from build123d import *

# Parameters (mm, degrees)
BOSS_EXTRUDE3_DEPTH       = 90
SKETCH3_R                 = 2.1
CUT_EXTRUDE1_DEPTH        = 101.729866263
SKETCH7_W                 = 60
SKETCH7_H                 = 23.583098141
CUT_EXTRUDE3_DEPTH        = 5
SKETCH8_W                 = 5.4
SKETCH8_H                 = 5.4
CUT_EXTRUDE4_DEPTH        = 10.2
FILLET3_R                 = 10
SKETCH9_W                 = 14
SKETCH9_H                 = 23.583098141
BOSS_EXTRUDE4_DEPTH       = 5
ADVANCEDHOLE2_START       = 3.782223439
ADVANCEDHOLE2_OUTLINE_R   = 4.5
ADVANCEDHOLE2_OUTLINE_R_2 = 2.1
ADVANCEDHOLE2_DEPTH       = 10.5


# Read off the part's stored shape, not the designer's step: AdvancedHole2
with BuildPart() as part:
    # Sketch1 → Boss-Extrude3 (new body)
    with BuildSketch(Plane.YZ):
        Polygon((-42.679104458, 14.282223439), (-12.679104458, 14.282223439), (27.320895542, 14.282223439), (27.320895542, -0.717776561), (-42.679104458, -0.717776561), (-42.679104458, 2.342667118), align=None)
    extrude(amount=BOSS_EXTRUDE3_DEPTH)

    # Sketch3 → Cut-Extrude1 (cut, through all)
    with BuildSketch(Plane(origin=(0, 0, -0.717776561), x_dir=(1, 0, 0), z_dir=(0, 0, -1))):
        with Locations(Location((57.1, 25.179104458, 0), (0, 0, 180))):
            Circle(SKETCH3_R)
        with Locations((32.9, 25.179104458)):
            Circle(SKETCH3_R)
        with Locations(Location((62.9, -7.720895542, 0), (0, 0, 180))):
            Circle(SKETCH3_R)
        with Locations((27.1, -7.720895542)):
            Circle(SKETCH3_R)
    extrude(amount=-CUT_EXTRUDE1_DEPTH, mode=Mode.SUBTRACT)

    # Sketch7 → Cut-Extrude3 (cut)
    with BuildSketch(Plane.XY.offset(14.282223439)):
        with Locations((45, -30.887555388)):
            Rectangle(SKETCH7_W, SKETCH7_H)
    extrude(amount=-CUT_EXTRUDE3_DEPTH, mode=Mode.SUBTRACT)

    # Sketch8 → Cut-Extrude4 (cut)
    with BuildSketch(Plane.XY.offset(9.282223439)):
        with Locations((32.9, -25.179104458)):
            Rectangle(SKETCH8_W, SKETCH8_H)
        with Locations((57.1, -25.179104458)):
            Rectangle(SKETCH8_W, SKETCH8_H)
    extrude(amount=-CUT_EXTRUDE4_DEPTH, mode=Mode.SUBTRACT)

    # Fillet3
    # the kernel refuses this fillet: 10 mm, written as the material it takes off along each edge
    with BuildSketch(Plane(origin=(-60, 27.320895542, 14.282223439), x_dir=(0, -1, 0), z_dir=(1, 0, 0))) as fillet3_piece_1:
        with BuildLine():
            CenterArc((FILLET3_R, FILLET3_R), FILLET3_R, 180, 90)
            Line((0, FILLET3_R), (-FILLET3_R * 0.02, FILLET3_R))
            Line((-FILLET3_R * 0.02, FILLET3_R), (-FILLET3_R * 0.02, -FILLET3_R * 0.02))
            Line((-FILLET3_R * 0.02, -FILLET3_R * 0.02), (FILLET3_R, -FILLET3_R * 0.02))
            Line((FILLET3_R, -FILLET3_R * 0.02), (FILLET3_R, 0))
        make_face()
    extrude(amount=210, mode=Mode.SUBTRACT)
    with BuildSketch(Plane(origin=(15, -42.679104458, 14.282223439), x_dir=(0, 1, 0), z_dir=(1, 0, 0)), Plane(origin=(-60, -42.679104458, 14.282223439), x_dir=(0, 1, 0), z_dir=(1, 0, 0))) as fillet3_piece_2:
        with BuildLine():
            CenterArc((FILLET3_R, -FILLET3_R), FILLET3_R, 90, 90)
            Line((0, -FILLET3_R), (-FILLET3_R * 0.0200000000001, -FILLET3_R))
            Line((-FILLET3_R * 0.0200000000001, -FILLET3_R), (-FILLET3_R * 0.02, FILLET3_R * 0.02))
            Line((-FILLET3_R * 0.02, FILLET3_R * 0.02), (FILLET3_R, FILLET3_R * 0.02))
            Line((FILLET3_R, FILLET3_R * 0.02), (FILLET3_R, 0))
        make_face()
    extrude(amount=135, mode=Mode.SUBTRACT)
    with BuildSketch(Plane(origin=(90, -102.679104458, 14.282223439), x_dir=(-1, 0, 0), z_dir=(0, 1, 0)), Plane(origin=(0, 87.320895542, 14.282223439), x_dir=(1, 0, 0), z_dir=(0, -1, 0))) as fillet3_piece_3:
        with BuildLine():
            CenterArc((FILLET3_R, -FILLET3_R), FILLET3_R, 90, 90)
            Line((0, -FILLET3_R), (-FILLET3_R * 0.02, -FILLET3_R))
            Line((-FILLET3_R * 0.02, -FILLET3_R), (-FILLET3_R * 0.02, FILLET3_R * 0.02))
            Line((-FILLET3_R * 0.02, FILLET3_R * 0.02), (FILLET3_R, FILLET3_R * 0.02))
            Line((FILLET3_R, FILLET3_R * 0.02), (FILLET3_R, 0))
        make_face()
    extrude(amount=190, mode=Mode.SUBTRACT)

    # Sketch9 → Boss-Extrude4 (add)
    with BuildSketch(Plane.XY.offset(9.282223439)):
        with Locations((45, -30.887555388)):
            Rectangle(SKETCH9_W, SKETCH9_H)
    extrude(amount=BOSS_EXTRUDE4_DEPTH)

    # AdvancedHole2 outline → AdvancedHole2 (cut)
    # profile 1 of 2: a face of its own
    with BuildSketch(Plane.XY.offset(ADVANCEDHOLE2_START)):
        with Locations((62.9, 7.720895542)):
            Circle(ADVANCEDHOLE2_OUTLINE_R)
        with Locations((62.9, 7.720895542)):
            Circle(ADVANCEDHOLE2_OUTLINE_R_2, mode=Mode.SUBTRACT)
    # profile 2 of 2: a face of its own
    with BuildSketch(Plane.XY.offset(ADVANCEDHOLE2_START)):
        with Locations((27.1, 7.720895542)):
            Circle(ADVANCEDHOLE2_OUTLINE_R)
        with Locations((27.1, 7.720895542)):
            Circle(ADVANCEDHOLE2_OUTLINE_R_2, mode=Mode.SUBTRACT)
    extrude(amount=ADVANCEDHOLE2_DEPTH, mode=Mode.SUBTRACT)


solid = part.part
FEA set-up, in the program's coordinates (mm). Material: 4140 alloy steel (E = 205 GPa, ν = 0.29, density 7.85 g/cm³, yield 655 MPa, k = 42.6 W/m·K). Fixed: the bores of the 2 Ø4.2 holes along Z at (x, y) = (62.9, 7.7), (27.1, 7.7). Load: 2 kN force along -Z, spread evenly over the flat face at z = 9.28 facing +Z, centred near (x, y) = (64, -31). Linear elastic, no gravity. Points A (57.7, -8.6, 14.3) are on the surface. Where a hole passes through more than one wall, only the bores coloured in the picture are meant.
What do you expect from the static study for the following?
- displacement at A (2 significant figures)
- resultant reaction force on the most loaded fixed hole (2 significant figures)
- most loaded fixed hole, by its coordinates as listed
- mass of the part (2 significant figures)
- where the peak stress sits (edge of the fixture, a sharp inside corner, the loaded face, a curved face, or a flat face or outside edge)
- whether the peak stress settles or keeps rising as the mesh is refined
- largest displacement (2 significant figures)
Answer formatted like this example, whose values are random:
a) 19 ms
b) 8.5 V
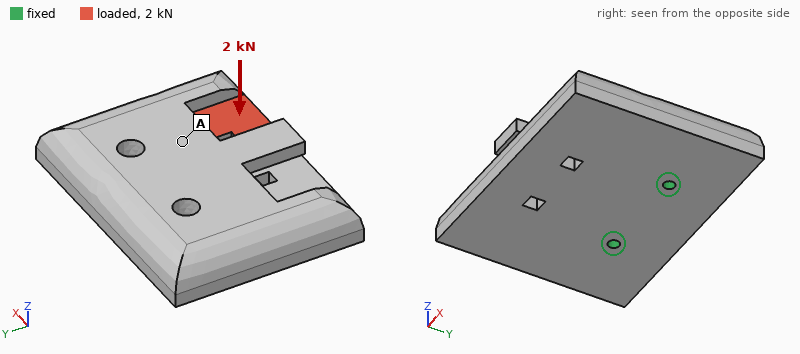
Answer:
a) 0.055 mm
b) 2.0 kN
c) (62.9, 7.7)
d) 640 g
e) edge of the fixture
f) keeps rising
g) 0.15 mm
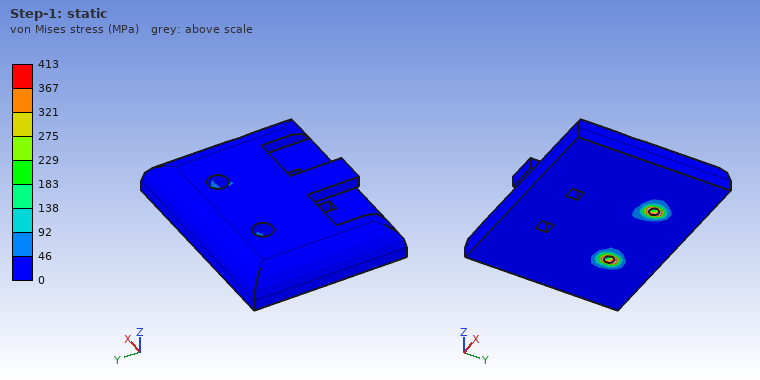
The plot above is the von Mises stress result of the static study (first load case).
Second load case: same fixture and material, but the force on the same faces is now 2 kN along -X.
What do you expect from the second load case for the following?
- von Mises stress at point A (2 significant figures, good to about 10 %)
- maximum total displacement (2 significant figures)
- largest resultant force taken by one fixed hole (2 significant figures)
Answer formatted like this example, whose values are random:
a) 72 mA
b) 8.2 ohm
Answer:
a) 7.3 MPa
b) 7.5 µm
c) 2.4 kN
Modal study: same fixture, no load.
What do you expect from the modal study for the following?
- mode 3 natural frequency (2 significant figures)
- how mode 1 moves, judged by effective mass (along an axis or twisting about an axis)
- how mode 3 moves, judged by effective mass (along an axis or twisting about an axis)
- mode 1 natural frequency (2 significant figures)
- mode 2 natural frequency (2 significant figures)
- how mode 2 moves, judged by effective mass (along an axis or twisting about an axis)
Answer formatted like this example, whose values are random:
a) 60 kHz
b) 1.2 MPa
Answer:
a) 5500 Hz
b) along Z
c) along X
d) 1400 Hz
e) 4200 Hz
f) twisting about Y
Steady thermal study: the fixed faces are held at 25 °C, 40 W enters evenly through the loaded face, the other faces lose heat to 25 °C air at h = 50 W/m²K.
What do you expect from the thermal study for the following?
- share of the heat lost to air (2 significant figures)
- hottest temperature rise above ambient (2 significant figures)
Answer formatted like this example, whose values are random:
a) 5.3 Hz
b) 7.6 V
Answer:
a) 44 %
b) 59 K
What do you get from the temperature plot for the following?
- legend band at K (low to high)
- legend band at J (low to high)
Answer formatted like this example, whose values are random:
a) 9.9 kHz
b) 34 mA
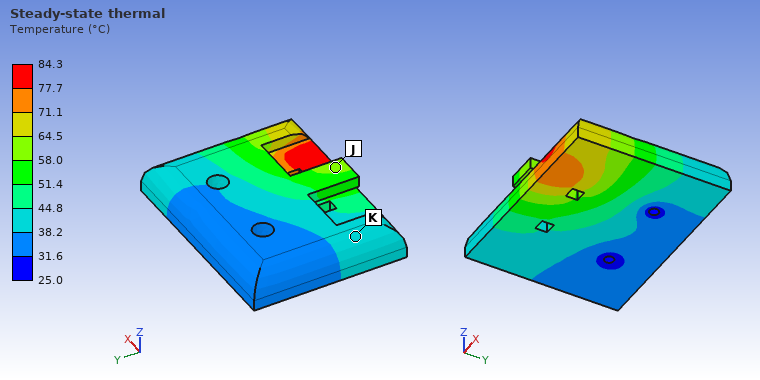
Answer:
a) 38.2 to 44.8 °C
b) 58.0 to 64.5 °C
